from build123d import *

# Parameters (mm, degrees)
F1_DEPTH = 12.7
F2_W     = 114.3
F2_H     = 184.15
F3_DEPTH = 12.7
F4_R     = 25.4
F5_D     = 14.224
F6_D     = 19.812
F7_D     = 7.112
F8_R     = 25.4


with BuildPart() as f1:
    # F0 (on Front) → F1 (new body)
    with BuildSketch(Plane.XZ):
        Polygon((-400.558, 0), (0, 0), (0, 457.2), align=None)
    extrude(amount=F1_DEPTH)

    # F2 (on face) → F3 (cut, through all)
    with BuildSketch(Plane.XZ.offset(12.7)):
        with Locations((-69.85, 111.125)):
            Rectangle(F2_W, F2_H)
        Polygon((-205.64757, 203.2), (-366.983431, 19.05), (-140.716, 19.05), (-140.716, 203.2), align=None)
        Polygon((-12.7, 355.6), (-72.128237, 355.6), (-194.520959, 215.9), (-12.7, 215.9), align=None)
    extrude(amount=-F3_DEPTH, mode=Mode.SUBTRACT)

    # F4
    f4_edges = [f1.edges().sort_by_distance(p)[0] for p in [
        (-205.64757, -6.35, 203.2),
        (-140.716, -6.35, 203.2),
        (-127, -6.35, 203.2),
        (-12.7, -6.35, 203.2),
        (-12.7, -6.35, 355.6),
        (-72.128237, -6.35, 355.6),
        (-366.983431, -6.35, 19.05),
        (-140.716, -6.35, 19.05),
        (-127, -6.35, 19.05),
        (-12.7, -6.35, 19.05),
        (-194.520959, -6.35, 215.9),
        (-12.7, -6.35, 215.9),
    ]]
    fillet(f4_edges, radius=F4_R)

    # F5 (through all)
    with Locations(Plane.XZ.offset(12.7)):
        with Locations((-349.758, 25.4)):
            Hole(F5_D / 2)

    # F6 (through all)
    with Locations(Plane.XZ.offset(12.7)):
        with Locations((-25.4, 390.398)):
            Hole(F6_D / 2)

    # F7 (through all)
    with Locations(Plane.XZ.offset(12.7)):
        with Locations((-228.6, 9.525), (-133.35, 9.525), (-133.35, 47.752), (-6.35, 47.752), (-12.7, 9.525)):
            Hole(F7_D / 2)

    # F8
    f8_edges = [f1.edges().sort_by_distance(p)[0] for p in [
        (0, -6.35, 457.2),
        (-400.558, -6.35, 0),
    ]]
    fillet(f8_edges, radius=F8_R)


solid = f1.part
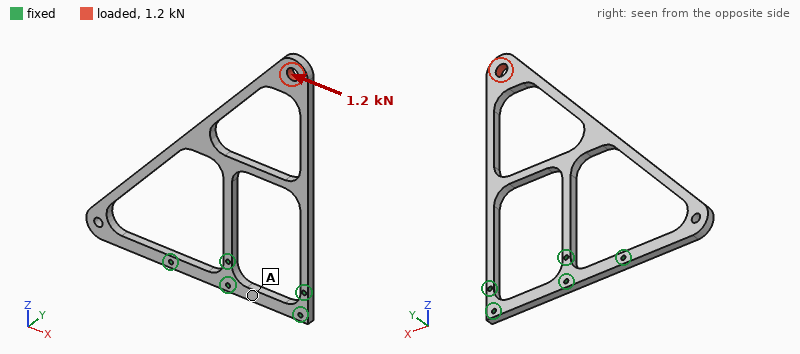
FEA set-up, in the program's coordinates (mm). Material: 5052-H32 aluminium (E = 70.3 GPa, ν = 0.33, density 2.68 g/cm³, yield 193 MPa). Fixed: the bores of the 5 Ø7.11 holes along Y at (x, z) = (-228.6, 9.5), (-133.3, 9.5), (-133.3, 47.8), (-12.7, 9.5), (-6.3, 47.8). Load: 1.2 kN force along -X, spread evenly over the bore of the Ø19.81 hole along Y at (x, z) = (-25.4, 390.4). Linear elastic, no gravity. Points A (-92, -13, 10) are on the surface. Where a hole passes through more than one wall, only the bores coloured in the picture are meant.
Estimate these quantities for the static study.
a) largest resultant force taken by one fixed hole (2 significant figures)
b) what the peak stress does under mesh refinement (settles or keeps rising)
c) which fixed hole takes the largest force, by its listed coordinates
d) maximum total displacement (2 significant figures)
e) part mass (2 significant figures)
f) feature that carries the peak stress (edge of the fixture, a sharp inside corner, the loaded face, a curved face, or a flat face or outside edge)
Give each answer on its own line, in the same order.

1.8 kN
keeps rising
(-6.3, 47.8)
1.3 mm
920 g
edge of the fixture
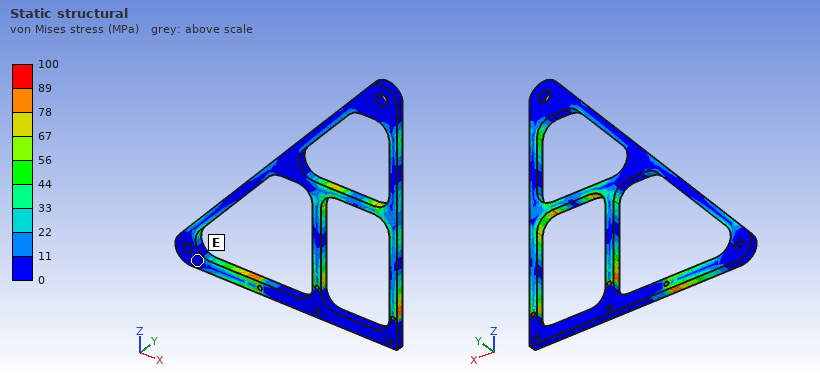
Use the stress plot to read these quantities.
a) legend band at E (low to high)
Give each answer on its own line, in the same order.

0 to 11 MPa
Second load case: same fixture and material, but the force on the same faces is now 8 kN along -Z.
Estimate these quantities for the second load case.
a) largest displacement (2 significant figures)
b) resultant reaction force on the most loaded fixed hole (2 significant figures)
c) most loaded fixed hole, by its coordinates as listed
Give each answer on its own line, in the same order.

0.56 mm
6.9 kN
(-6.3, 47.8)
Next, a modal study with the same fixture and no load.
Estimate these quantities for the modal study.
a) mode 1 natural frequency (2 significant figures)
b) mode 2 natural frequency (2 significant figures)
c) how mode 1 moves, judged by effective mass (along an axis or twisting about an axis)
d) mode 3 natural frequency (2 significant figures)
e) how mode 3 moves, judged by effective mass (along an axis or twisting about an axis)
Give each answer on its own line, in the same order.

65 Hz
200 Hz
along Y
240 Hz
along X
